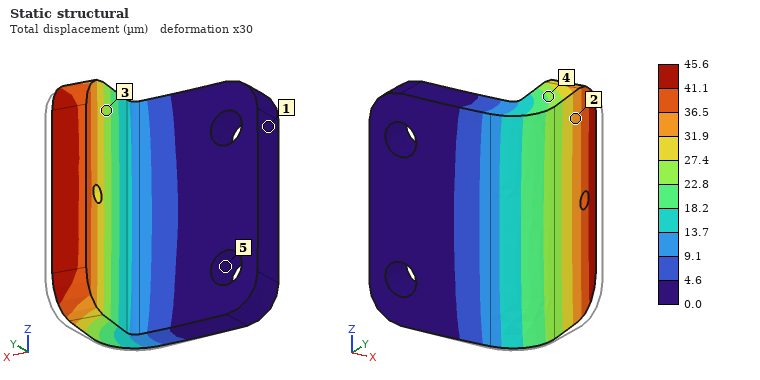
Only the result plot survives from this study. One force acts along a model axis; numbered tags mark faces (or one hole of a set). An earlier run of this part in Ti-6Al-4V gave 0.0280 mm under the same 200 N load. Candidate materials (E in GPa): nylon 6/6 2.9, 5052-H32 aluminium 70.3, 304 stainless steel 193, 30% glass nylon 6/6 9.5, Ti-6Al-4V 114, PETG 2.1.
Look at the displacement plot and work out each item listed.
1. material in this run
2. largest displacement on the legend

5052-H32 aluminium
45.6 µm
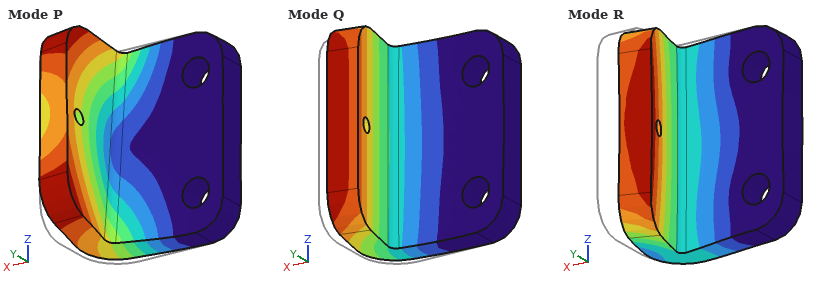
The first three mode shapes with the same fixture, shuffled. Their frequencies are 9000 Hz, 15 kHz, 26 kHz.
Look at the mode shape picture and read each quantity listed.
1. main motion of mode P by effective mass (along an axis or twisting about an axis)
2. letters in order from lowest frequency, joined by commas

along Z
Q, P, R
